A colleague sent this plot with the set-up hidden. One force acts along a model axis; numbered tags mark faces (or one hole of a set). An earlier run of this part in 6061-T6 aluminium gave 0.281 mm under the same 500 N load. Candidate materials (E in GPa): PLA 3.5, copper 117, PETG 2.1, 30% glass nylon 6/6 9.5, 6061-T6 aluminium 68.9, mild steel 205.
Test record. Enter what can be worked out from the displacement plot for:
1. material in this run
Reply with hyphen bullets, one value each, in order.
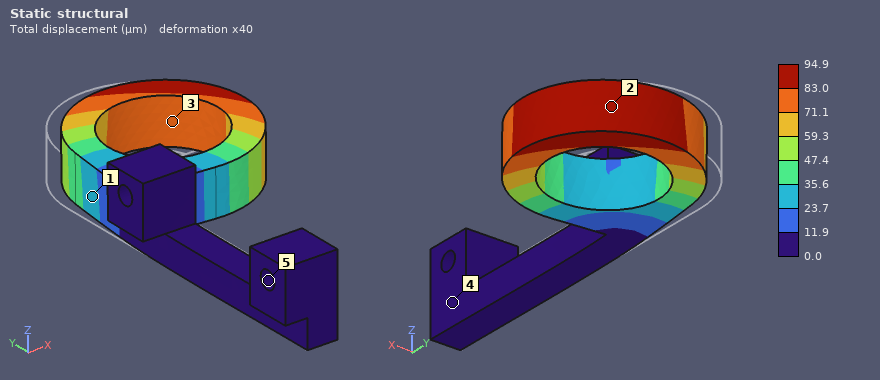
- mild steel
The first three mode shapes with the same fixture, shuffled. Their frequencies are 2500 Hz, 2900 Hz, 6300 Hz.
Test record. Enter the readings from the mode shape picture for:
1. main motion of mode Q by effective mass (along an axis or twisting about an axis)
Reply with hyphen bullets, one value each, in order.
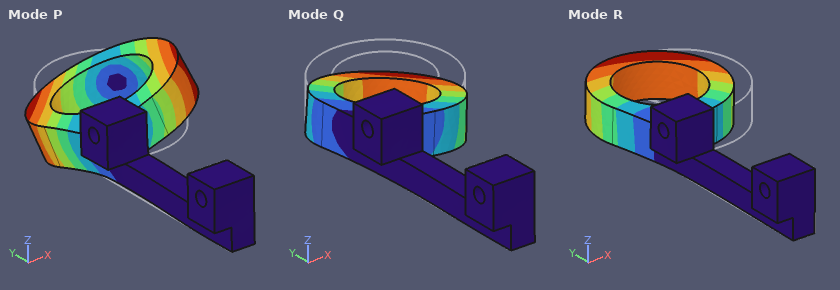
- along Z
